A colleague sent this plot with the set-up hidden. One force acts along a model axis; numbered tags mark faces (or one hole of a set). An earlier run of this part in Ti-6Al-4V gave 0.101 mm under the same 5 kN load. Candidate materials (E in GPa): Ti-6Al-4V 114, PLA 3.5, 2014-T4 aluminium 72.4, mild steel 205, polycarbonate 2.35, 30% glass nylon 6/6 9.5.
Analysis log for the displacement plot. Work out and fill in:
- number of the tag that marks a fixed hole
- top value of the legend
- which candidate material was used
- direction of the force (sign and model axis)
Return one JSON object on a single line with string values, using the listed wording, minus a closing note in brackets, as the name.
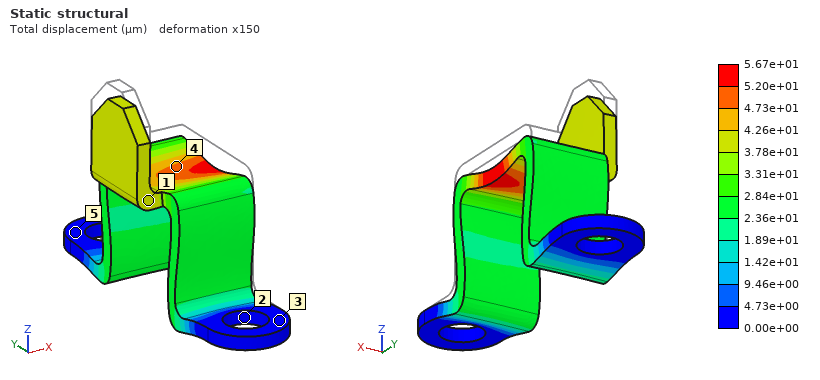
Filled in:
{"number of the tag that marks a fixed hole": "2", "top value of the legend": "5.67e+01 µm", "which candidate material was used": "mild steel", "direction of the force": "-Z"}
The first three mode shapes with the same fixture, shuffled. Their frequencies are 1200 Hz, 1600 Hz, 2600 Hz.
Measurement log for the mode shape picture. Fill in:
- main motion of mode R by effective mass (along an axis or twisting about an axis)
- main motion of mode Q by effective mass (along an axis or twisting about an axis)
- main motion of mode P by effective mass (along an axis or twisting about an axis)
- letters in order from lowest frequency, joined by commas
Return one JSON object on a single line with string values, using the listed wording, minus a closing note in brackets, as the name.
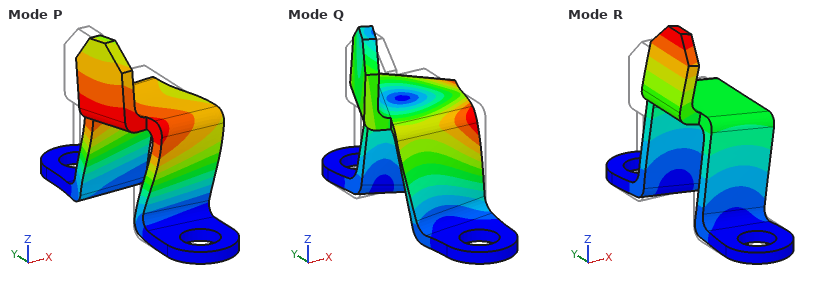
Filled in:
{"main motion of mode R by effective mass": "along X", "main motion of mode Q by effective mass": "twisting about Z", "main motion of mode P by effective mass": "along Y", "letters in order from lowest frequency, joined by commas": "R, P, Q"}
